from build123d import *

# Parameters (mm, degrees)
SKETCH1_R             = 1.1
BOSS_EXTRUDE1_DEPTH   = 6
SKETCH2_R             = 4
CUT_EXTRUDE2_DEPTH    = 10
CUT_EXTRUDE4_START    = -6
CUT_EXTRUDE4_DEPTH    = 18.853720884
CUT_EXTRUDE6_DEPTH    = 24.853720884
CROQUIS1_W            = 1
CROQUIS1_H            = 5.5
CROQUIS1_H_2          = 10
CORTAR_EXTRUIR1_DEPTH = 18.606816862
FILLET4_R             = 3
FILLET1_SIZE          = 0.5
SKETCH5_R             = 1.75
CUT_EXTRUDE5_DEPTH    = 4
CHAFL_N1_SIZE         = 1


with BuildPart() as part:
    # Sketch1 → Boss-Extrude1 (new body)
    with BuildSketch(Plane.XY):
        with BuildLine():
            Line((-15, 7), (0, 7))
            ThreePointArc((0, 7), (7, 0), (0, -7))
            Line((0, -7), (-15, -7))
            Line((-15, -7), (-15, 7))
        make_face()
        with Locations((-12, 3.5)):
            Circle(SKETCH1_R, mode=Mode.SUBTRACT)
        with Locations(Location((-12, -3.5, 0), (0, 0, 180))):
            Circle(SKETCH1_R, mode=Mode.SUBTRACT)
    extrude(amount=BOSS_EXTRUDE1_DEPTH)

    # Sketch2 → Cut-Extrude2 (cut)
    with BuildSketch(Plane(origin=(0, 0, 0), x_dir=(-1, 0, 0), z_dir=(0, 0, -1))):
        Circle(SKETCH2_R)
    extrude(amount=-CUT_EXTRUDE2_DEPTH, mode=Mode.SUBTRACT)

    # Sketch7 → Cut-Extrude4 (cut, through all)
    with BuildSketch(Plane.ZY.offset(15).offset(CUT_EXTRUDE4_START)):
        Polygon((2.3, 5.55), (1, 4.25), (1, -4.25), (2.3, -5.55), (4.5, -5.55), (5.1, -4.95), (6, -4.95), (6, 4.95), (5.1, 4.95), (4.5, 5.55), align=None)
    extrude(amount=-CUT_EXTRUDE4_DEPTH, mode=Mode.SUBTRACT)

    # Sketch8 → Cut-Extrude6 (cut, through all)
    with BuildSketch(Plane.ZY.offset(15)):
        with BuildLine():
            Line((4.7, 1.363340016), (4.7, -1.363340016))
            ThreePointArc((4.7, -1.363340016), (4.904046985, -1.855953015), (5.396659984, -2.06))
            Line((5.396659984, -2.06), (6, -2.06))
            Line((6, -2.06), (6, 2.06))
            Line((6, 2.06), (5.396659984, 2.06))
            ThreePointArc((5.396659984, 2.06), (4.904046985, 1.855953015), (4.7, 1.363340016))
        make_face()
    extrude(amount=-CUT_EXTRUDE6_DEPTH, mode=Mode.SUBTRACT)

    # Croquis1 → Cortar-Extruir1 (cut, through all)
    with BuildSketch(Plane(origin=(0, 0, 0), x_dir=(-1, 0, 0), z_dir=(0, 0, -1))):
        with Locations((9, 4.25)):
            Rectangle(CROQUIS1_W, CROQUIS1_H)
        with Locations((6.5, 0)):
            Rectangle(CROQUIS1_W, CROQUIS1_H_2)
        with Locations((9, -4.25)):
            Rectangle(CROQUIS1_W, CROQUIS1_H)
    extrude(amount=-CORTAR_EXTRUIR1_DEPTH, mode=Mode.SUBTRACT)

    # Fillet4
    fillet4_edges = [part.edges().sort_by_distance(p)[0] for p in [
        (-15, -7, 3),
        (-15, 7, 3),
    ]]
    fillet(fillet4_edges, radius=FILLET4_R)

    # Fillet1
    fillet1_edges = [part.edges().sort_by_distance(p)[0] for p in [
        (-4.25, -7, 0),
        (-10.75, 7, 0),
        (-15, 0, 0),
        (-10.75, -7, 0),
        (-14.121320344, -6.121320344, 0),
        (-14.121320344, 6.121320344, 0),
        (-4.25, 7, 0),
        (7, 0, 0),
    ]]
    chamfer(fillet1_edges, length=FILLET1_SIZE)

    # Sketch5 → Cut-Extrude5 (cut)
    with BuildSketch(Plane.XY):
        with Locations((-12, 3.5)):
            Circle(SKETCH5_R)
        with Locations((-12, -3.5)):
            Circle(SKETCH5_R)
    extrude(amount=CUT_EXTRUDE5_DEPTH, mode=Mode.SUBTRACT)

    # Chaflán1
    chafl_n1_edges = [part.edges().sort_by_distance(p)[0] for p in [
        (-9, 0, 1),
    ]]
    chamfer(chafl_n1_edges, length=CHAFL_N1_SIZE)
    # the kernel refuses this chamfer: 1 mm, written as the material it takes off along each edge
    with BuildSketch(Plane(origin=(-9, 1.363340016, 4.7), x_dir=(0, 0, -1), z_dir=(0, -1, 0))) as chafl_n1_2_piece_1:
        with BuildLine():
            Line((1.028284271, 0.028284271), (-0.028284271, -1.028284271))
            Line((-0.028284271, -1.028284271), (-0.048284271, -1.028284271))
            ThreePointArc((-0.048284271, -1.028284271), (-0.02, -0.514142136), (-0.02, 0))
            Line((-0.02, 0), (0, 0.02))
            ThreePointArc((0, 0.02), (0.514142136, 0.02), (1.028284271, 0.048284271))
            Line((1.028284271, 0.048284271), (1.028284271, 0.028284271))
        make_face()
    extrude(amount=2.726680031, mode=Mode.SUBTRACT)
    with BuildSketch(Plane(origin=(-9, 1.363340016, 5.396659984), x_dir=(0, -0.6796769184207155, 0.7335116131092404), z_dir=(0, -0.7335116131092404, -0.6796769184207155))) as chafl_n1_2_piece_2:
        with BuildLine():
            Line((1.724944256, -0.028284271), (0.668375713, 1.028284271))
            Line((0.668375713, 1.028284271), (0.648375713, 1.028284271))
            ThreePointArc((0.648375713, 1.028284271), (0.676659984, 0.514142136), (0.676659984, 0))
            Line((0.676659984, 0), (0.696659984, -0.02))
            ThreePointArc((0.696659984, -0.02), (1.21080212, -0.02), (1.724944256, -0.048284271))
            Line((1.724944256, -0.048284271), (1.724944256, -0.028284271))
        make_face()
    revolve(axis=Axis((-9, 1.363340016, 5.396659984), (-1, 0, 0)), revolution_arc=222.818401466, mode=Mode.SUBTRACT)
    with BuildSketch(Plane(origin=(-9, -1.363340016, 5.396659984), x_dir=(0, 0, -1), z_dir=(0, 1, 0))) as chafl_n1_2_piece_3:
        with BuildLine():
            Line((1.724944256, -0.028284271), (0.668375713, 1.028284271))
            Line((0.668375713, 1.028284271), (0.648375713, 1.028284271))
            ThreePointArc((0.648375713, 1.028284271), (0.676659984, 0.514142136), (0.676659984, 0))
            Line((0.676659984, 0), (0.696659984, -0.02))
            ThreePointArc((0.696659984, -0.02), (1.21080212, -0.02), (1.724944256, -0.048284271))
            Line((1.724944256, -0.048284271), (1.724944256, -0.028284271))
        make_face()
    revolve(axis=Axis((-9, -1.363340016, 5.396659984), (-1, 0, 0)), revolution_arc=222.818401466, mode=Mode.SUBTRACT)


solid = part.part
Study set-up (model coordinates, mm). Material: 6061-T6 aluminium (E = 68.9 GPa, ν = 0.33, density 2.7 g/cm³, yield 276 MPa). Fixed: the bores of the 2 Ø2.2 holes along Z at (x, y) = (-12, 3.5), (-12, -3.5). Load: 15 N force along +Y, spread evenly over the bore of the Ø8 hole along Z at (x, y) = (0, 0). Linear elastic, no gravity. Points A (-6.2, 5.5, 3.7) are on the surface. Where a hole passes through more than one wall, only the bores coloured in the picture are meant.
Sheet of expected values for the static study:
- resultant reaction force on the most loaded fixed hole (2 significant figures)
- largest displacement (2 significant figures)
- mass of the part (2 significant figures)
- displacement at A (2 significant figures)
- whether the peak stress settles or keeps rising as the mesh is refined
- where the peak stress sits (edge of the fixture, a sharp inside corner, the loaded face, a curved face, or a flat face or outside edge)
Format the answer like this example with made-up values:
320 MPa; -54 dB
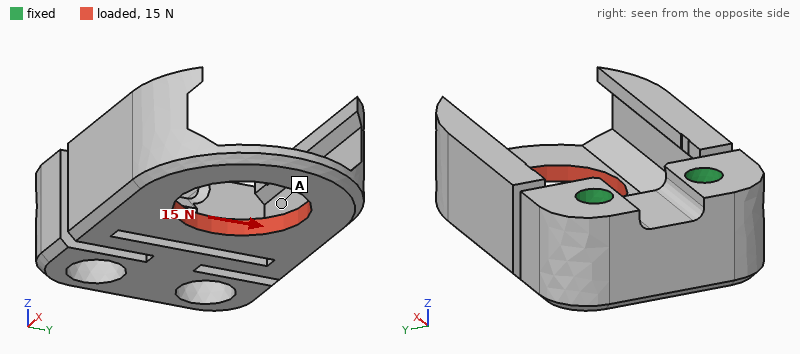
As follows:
22 N; 77 µm; 1.8 g; 29 µm; keeps rising; a sharp inside corner
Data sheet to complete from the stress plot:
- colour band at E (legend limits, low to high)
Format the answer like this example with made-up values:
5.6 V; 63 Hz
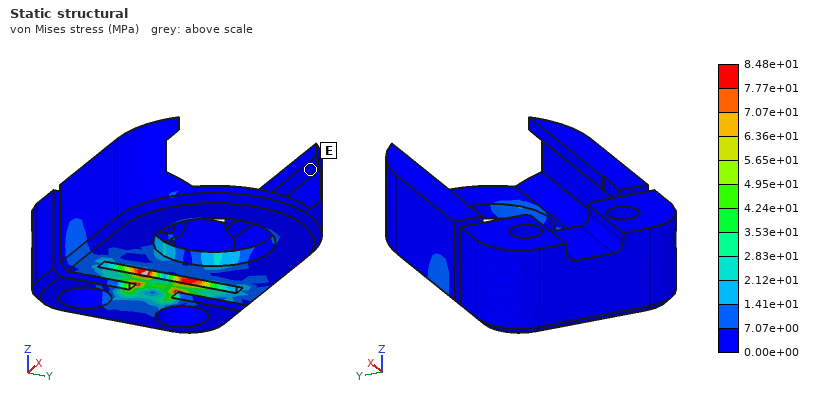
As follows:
0.00e+00 to 7.07e+00 MPa
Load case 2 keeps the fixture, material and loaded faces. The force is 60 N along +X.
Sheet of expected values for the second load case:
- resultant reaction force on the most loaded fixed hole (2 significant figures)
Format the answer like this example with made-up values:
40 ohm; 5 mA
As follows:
30 N
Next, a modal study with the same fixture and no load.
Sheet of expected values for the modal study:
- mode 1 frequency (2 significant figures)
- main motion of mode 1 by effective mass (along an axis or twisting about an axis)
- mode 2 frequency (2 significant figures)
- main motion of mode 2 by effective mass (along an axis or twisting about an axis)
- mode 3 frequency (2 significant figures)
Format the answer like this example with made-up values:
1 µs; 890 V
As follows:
1400 Hz; along Z; 2600 Hz; along Y; 3500 Hz
